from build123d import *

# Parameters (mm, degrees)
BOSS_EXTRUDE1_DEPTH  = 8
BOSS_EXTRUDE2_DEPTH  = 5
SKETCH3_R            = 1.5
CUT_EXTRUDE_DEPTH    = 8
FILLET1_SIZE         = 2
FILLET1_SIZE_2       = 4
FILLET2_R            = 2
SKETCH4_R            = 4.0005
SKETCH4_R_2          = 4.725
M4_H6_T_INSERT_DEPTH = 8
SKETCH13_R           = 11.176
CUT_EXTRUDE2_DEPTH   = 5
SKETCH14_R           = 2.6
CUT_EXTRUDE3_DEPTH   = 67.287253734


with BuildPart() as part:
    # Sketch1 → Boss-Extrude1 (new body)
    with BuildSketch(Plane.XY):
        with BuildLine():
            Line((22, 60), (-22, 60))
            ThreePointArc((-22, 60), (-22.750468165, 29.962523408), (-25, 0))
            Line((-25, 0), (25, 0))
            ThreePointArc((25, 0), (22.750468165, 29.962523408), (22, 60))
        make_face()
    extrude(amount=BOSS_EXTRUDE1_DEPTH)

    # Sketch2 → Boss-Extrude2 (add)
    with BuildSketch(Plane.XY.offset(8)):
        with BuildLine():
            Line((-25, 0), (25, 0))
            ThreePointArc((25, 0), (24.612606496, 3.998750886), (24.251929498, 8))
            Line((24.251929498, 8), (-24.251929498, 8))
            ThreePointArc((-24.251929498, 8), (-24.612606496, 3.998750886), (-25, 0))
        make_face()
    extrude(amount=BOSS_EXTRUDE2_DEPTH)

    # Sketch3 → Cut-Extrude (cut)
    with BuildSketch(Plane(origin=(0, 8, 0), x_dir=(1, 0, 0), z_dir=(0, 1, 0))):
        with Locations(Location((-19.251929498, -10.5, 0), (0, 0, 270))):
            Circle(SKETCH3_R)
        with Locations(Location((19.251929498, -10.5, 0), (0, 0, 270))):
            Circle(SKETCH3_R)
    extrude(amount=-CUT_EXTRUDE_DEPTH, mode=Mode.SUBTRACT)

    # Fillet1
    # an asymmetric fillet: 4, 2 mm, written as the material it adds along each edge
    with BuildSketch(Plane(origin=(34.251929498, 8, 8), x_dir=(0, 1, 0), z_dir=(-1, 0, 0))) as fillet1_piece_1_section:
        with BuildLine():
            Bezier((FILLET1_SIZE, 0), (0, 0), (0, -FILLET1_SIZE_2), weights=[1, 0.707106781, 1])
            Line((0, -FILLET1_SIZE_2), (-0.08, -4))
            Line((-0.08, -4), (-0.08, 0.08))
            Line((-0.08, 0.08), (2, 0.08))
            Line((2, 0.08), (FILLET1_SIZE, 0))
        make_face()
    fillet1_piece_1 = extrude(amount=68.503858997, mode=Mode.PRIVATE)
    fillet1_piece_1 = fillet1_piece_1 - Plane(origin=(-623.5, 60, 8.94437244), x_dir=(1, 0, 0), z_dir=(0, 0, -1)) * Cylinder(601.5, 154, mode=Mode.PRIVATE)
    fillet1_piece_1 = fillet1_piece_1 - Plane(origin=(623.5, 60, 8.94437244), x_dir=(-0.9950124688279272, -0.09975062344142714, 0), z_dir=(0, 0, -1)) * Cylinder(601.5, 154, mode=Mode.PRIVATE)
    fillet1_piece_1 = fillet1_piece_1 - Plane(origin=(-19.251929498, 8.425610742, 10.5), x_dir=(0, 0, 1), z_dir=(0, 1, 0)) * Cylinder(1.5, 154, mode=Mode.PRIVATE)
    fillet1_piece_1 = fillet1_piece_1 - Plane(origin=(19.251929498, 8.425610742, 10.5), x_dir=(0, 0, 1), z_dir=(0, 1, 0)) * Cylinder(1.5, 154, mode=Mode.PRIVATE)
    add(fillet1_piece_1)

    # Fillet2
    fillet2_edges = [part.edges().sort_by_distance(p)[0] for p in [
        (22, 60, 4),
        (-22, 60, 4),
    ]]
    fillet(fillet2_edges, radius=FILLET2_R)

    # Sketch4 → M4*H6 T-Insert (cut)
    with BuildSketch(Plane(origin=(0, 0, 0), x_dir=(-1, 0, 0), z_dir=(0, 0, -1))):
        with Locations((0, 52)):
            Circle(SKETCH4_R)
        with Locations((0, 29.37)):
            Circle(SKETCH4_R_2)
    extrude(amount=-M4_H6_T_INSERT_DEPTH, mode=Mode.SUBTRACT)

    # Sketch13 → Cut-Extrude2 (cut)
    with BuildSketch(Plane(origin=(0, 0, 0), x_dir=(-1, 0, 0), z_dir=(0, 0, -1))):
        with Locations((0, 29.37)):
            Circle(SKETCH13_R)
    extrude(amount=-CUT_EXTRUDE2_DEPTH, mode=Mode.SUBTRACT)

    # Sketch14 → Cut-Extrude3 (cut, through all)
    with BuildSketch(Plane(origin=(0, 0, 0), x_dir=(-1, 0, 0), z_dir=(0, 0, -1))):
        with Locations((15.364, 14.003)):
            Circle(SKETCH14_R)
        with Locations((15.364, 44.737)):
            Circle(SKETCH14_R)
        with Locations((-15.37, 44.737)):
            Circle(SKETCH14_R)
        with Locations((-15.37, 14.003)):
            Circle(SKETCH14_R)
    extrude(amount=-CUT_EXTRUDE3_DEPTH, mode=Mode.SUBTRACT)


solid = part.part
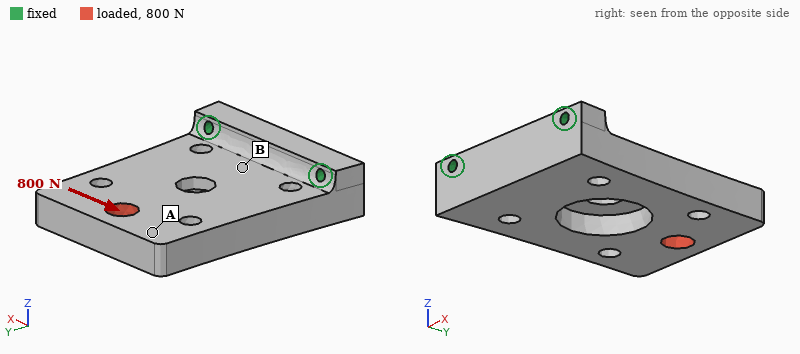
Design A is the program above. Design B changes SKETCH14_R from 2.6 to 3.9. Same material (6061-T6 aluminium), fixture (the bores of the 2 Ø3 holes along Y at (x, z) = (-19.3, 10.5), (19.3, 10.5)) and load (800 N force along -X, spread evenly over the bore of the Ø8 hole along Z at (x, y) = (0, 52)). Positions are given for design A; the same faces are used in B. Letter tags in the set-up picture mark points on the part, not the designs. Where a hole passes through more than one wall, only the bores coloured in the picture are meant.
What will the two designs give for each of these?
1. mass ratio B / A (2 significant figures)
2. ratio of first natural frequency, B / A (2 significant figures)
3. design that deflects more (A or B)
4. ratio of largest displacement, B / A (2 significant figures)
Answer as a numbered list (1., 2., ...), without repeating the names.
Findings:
1. 0.96
2. 0.97
3. B
4. 1.1
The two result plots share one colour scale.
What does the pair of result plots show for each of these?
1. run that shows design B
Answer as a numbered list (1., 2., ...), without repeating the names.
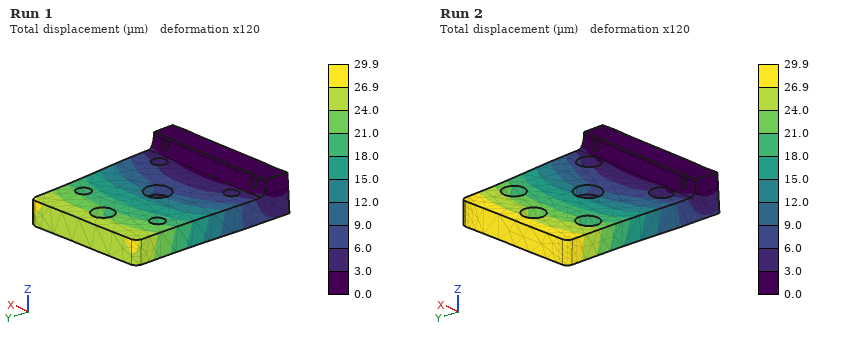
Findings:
1. Run 2
